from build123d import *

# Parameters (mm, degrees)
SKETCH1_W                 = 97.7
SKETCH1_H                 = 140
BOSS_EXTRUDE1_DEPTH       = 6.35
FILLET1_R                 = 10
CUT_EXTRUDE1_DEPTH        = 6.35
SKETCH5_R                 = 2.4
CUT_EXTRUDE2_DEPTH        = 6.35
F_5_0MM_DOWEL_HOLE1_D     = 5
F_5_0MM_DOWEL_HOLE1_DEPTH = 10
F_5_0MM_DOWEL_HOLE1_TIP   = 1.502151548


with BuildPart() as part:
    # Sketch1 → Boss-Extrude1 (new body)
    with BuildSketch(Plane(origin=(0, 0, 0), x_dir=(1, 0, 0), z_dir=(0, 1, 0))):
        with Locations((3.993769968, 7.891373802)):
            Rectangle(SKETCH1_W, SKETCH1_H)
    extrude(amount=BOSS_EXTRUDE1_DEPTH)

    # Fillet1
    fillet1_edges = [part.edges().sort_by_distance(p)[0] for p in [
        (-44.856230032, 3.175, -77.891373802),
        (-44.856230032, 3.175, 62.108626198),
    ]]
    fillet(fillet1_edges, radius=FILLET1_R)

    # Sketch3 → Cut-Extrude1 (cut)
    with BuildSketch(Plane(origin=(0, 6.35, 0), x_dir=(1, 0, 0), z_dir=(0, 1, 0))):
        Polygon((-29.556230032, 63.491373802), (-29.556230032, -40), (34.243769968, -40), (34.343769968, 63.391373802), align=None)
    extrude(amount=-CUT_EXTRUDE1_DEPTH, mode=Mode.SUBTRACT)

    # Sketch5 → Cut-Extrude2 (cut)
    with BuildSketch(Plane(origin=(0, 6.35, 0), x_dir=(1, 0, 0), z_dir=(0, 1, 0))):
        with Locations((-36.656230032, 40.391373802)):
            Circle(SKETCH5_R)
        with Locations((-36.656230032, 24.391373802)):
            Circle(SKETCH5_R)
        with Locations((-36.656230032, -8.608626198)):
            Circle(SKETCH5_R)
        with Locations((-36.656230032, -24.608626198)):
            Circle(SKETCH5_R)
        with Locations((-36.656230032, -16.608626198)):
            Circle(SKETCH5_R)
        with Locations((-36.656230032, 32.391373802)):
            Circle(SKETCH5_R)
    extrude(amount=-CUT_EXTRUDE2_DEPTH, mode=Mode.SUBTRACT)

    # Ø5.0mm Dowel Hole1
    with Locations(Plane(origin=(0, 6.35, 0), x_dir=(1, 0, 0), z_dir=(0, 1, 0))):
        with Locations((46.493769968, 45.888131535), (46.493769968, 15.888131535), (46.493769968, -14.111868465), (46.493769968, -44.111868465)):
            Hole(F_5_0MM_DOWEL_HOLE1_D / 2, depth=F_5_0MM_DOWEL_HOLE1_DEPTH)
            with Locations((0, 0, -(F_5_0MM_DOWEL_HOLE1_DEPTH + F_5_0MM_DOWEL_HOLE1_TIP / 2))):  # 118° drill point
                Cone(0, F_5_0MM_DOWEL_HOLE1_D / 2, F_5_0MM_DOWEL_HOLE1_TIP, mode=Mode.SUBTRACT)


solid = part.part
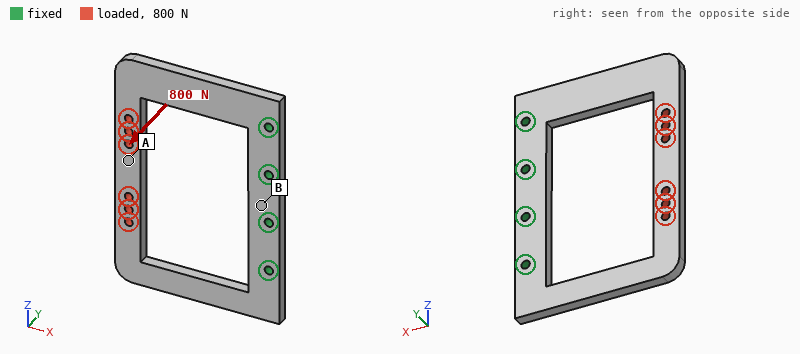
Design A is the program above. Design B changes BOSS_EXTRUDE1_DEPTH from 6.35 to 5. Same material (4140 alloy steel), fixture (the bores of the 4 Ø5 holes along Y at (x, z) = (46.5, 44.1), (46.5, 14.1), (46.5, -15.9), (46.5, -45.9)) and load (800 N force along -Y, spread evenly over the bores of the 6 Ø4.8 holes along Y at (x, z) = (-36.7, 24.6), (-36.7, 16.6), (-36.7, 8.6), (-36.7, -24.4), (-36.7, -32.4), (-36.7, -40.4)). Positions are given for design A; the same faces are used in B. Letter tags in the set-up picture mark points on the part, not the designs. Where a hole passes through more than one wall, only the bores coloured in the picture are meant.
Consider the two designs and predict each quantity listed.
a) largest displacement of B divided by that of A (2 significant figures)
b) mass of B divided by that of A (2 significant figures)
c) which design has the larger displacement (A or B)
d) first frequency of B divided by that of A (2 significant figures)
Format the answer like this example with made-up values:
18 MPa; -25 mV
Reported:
2.0; 0.79; B; 0.80
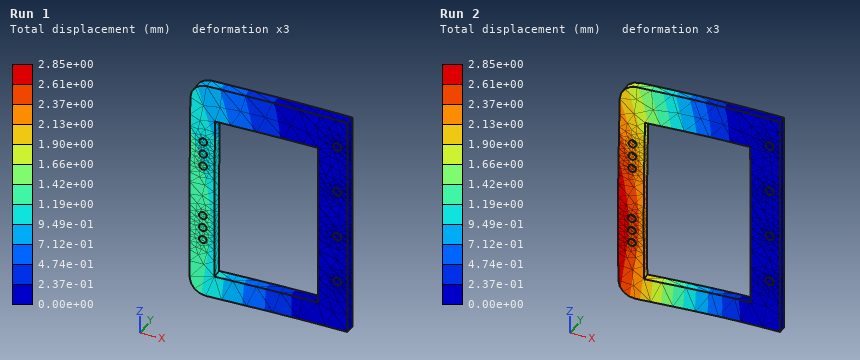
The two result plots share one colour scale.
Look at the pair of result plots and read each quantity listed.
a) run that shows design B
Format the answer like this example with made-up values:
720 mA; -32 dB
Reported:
Run 2
